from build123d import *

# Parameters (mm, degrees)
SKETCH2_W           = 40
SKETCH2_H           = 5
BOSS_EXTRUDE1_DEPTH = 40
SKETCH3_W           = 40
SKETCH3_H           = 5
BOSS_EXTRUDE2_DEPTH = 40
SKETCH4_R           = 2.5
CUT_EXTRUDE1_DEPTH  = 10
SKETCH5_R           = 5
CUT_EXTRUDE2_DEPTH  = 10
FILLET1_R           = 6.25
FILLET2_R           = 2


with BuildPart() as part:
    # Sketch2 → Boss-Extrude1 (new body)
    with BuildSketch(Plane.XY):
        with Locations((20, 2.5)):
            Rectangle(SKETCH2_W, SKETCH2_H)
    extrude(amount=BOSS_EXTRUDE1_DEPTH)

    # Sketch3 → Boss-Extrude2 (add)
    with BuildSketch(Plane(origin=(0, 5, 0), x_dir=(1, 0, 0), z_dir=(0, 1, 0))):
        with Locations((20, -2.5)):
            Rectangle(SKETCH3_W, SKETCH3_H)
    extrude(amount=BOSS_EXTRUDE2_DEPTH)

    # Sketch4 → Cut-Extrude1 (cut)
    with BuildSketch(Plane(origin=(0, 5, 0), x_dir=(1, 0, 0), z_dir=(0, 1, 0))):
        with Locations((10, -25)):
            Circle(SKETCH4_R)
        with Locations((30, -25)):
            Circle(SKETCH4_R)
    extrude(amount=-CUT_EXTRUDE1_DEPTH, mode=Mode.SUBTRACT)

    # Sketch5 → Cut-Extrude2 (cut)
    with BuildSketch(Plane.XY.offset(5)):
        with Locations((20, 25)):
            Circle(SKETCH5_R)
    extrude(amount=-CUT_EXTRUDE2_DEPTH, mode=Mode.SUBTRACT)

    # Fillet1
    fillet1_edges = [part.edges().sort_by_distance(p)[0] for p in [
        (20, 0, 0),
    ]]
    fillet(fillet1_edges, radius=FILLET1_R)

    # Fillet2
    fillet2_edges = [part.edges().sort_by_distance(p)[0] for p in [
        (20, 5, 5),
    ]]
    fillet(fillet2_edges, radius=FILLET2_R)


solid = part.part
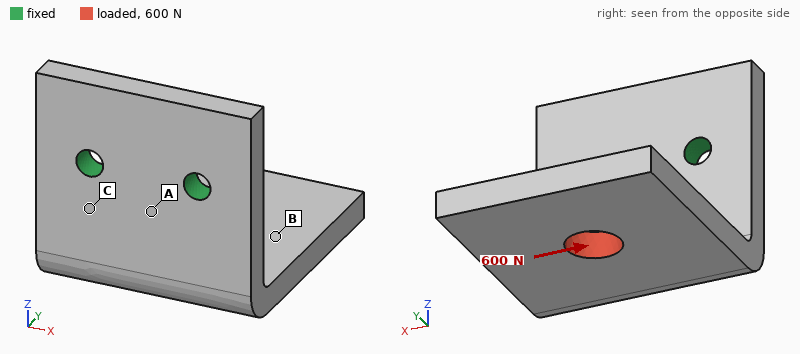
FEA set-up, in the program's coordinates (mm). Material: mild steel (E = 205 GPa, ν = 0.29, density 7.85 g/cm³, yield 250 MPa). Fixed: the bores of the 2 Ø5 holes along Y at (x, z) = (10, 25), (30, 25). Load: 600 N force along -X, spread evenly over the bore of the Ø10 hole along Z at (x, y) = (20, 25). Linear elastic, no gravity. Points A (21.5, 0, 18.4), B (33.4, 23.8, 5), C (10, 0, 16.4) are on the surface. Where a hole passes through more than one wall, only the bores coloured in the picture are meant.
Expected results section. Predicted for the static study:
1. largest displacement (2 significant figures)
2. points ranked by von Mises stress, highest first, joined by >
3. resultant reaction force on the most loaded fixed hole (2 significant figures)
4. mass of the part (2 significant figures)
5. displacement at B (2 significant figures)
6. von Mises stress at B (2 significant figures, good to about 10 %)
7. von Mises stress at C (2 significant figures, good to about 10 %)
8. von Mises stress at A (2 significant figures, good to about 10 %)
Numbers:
57 µm
C > A > B
810 N
120 g
31 µm
10 MPa
37 MPa
24 MPa
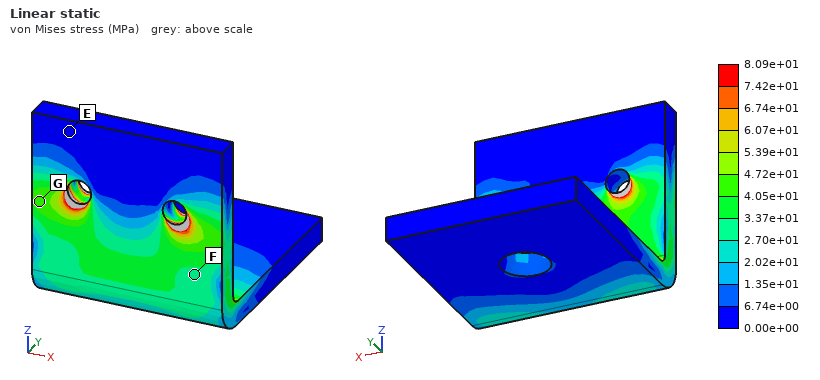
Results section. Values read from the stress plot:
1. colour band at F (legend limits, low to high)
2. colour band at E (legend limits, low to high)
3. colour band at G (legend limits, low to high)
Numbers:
2.70e+01 to 3.37e+01 MPa
0.00e+00 to 6.74e+00 MPa
4.05e+01 to 4.72e+01 MPa
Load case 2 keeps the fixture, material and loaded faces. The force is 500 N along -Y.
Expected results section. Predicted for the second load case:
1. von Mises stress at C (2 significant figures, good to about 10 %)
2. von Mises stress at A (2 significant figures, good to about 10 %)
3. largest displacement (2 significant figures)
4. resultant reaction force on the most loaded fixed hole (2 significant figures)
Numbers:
40 MPa
38 MPa
64 µm
250 N
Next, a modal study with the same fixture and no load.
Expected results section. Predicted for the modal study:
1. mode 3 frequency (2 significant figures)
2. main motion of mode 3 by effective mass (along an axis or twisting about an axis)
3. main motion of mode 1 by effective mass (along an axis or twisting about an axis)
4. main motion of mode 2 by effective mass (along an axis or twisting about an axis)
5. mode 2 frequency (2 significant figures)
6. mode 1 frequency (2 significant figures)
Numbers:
4300 Hz
along Y
along Z
along X
2400 Hz
1300 Hz
